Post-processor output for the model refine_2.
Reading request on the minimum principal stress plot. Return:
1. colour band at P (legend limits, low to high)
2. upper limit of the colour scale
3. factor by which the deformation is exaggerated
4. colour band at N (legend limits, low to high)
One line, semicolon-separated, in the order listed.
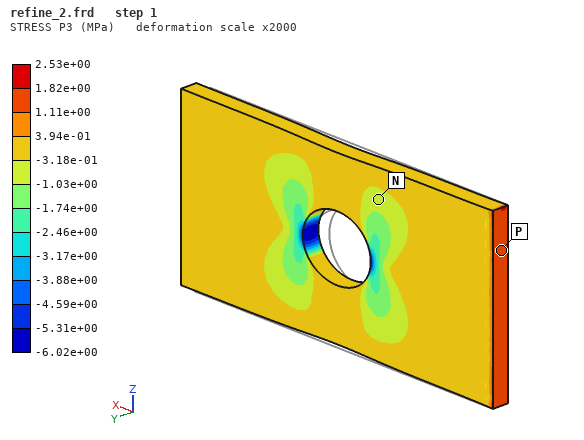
1.11e+00 to 1.82e+00 MPa; 2.53e+00 MPa; 2000; -1.03e+00 to -3.18e-01 MPa
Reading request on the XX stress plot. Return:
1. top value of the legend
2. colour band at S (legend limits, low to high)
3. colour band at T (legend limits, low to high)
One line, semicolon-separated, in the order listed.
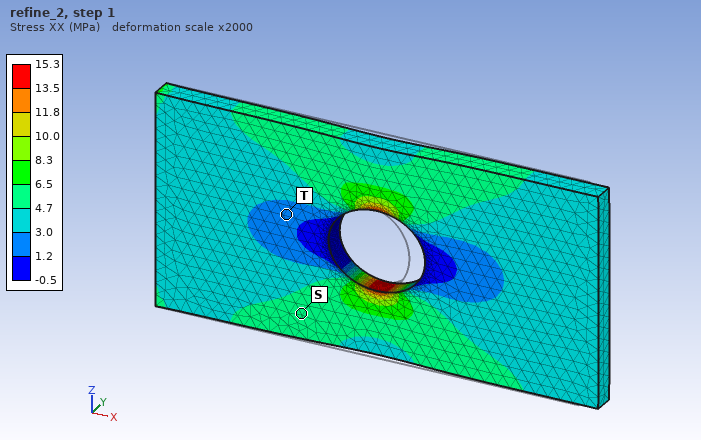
15.3 MPa; 4.7 to 6.5 MPa; 1.2 to 3.0 MPa
